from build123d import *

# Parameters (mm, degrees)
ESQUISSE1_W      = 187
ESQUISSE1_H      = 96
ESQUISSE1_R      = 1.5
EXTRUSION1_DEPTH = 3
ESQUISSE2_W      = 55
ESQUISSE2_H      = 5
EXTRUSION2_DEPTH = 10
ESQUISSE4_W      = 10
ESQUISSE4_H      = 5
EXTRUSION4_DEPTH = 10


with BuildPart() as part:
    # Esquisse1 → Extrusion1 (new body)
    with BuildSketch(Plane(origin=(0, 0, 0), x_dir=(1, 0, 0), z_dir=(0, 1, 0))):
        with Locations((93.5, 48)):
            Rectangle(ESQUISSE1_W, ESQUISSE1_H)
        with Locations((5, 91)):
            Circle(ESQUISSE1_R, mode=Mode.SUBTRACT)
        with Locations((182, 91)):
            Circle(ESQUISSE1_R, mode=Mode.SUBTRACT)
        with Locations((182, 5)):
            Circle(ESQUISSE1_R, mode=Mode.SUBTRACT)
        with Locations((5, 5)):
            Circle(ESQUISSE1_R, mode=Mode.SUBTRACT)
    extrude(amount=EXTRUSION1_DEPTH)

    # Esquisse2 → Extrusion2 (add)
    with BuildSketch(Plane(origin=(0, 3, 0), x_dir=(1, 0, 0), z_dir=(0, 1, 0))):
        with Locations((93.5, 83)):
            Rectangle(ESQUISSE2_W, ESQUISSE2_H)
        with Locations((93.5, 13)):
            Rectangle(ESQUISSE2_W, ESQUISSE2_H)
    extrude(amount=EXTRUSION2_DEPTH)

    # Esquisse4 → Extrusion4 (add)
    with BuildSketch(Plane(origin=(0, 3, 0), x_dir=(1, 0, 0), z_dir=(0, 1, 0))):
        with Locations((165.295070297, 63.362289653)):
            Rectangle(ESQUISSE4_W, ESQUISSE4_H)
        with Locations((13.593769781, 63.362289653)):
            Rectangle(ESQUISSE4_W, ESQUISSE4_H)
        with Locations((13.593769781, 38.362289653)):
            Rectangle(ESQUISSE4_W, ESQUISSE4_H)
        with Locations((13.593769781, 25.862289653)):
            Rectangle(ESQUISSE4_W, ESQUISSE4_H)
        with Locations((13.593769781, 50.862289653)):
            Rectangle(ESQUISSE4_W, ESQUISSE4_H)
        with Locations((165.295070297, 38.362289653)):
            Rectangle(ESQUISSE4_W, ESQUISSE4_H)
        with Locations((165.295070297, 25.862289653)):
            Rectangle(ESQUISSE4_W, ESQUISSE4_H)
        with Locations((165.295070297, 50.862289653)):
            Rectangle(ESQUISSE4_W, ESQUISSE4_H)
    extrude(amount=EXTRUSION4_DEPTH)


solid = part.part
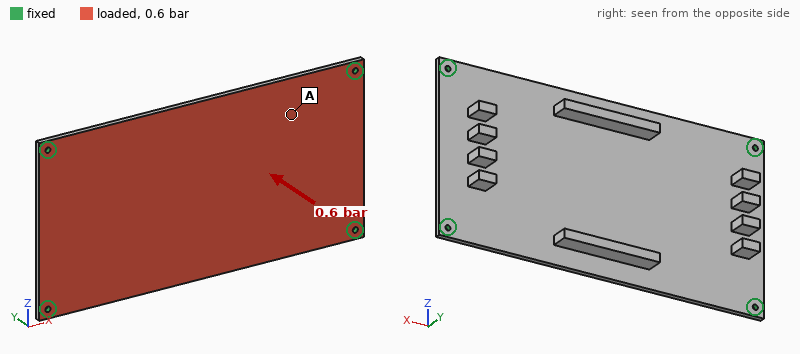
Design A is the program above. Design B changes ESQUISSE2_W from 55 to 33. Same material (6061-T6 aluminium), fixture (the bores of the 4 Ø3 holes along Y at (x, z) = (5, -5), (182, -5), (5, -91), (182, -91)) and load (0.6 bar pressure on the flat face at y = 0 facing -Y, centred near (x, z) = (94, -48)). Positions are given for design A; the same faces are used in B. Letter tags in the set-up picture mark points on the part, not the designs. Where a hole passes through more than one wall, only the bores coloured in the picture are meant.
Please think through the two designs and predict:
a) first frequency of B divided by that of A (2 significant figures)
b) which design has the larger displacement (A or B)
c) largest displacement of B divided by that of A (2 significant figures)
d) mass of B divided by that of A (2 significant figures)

0.91
B
1.3
0.97
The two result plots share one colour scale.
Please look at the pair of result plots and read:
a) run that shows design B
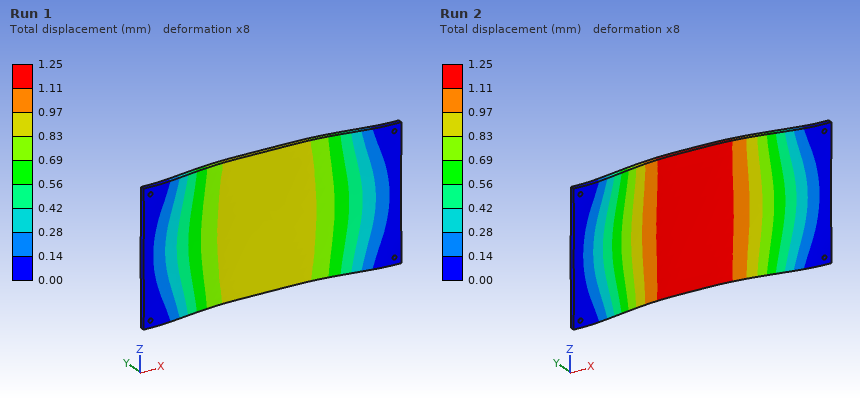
Run 2
